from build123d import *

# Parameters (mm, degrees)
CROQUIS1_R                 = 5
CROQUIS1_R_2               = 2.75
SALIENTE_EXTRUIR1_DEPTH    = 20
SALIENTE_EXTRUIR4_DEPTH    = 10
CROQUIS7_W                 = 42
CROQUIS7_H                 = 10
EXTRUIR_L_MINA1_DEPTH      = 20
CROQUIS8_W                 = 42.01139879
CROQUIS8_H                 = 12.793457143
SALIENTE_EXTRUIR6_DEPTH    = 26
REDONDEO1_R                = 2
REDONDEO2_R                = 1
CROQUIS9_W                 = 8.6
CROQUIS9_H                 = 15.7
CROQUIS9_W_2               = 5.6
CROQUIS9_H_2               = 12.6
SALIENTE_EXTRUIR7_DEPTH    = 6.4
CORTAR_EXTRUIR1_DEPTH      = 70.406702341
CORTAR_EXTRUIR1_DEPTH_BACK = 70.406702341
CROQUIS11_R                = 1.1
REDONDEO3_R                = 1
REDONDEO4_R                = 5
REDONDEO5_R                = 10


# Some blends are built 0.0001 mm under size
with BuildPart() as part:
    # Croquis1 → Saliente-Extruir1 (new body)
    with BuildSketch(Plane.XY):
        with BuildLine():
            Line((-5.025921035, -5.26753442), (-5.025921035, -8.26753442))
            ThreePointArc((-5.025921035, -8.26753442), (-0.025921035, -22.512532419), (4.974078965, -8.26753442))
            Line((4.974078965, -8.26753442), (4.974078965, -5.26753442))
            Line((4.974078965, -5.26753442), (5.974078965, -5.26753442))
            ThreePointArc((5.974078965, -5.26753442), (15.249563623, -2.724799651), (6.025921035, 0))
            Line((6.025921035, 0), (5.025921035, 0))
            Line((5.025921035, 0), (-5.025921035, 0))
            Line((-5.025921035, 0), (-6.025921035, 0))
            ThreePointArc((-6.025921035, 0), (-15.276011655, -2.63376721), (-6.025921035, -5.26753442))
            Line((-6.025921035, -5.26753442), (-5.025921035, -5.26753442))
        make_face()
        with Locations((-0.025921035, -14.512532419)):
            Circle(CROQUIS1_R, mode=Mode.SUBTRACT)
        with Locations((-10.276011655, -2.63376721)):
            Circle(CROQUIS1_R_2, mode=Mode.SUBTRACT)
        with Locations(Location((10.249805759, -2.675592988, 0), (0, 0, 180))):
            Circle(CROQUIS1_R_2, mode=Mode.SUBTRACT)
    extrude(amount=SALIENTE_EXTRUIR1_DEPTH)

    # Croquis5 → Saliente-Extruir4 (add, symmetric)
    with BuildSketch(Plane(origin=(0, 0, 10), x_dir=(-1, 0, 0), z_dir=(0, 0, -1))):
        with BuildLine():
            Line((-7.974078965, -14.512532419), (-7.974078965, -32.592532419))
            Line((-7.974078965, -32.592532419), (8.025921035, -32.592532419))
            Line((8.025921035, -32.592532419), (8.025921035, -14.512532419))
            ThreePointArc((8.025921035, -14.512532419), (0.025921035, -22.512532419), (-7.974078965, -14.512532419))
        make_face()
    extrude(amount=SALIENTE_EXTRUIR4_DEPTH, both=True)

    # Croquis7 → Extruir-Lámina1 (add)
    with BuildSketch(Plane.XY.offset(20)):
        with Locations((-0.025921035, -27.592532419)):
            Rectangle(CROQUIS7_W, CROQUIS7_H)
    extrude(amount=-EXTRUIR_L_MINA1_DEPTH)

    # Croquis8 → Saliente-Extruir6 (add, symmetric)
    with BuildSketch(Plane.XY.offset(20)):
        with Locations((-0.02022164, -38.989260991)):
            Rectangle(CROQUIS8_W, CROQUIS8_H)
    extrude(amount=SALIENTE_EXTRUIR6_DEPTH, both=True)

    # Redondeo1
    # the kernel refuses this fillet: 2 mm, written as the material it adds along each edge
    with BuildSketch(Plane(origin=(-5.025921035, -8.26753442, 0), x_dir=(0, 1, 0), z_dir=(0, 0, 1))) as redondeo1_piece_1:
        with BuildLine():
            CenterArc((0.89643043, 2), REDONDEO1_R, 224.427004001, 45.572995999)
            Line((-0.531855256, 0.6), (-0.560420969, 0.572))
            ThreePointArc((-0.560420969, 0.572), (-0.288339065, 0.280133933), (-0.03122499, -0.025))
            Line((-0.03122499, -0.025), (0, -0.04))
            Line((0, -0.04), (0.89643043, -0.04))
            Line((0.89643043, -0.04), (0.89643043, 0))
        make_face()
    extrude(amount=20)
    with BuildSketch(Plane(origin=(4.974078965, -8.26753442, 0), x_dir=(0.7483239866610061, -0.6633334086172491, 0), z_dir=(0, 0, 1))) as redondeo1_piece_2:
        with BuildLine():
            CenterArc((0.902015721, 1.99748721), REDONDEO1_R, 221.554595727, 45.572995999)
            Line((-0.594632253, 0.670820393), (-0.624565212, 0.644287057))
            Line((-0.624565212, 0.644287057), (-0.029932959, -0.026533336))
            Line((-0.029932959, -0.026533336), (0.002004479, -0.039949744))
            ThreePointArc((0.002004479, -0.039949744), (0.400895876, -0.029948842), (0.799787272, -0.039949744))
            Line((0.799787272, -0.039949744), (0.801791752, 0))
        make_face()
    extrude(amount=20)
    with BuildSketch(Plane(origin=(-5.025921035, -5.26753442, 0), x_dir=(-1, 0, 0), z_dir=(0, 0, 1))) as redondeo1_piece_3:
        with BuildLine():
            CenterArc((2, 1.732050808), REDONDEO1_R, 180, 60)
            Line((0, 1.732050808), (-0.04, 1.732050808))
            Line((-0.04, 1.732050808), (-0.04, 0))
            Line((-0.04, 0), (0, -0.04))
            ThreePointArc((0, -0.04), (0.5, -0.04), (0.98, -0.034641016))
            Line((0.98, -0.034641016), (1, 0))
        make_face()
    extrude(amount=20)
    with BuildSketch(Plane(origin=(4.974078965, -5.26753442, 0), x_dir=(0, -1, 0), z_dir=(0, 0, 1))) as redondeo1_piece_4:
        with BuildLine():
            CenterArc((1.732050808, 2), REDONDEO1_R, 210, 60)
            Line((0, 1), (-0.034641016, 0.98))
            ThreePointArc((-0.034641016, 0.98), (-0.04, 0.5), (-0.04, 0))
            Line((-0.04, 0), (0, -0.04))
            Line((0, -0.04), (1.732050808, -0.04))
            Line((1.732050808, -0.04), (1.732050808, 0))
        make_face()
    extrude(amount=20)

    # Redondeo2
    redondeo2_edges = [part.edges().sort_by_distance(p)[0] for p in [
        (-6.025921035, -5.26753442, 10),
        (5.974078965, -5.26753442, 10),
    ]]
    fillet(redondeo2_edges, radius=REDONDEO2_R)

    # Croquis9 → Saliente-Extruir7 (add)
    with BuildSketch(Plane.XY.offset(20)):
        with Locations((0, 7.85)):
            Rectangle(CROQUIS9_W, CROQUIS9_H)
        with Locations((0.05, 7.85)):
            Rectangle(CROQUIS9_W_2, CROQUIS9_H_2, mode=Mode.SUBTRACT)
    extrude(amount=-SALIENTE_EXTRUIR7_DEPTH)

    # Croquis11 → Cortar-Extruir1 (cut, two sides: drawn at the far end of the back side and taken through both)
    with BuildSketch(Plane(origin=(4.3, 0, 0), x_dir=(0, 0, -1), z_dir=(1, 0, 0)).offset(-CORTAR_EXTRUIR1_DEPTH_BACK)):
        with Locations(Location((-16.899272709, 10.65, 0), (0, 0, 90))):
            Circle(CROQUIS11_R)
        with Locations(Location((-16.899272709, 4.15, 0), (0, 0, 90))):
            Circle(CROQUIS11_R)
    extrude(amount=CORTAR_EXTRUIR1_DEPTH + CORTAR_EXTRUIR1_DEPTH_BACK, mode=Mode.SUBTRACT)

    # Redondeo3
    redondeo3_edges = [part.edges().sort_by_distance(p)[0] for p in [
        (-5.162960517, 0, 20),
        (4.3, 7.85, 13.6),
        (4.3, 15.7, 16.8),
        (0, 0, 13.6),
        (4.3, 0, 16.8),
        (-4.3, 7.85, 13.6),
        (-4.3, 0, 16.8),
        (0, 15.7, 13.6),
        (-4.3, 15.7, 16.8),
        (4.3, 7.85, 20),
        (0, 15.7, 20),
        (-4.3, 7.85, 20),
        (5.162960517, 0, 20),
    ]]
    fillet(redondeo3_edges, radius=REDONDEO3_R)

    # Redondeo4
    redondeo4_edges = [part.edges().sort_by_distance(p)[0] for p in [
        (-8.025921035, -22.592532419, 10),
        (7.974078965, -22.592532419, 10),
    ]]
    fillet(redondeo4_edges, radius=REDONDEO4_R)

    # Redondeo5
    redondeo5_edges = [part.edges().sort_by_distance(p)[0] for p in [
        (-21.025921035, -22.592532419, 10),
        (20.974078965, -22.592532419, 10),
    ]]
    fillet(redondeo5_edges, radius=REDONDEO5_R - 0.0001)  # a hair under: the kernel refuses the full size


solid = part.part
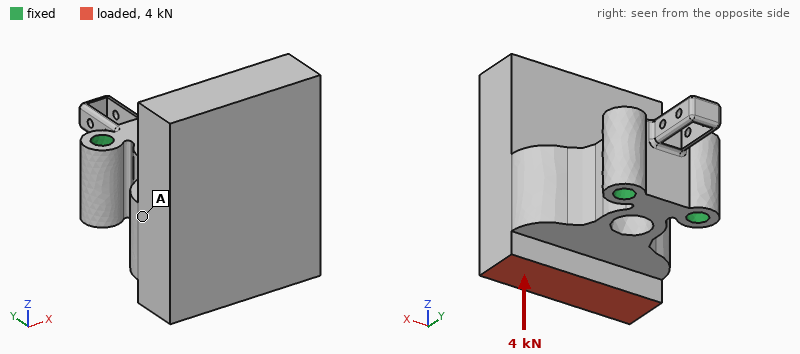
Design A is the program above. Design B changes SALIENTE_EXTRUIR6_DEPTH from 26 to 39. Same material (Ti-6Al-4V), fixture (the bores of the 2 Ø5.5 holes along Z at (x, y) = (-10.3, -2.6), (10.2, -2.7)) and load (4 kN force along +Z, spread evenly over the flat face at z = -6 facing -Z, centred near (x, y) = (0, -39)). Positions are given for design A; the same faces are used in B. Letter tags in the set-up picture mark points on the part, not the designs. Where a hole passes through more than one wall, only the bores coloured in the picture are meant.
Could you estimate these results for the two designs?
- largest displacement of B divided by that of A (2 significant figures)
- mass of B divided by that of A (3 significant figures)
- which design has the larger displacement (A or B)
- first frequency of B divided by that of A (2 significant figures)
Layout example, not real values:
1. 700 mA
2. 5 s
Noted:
1. 1.2
2. 1.33
3. B
4. 0.83
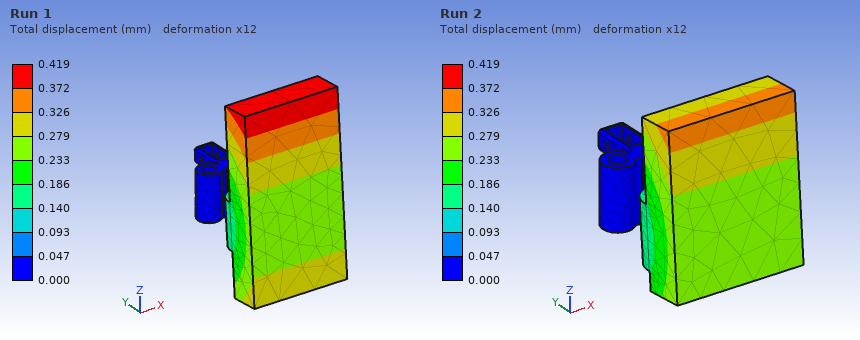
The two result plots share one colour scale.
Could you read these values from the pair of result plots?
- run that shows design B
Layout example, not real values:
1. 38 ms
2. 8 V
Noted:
1. Run 1
